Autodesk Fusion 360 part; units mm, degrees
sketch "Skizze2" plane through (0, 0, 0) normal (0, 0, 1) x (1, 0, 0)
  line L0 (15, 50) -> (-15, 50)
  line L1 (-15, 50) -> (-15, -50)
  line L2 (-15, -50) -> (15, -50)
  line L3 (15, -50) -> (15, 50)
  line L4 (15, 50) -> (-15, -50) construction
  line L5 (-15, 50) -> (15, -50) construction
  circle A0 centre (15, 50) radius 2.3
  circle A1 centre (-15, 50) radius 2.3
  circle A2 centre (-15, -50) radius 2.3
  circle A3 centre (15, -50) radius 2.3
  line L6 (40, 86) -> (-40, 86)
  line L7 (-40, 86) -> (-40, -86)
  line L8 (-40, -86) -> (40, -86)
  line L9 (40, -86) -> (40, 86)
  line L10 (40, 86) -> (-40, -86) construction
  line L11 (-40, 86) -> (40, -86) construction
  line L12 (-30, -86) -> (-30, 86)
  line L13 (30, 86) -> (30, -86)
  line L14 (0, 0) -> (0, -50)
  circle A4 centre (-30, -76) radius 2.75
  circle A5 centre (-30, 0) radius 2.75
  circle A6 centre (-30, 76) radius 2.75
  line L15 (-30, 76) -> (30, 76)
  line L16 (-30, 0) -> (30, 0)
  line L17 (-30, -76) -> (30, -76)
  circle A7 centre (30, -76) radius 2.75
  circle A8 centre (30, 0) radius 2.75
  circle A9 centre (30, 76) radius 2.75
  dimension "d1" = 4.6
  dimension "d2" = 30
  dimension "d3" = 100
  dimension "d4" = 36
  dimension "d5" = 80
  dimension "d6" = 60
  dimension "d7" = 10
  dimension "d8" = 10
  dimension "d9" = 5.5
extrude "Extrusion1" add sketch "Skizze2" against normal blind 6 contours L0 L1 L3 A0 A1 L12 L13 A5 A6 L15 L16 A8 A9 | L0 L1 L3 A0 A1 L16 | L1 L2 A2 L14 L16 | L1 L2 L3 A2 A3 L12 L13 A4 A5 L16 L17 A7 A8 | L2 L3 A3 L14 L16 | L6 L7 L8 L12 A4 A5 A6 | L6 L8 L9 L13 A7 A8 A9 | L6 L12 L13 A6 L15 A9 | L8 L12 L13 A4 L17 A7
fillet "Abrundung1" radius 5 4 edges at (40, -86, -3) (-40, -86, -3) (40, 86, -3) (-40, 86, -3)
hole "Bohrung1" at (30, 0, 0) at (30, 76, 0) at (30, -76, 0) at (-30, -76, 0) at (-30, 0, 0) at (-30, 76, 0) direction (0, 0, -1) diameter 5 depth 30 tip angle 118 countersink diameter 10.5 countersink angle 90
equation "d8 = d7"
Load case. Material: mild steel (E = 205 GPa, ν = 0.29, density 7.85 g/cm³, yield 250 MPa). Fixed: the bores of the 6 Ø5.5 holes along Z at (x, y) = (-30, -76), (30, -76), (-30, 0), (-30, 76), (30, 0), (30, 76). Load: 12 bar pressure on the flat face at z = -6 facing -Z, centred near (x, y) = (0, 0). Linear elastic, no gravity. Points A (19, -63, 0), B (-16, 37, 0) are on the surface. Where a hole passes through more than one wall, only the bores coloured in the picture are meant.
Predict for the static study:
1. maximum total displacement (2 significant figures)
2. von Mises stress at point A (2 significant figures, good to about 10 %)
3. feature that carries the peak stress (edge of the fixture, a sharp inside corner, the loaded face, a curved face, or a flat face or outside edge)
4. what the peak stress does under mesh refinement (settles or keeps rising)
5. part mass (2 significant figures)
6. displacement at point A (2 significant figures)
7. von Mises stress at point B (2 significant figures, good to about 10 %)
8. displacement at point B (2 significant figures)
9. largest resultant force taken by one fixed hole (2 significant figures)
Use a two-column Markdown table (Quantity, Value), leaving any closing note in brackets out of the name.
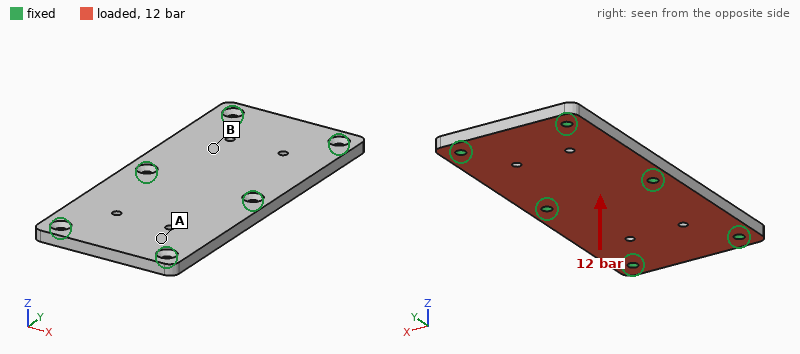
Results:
| Quantity | Value |
|---|---|
| maximum total displacement | 56 µm |
| von Mises stress at point A | 25 MPa |
| feature that carries the peak stress | edge of the fixture |
| what the peak stress does under mesh refinement | keeps rising |
| part mass | 630 g |
| displacement at point A | 28 µm |
| von Mises stress at point B | 50 MPa |
| displacement at point B | 50 µm |
| largest resultant force taken by one fixed hole | 4.0 kN |
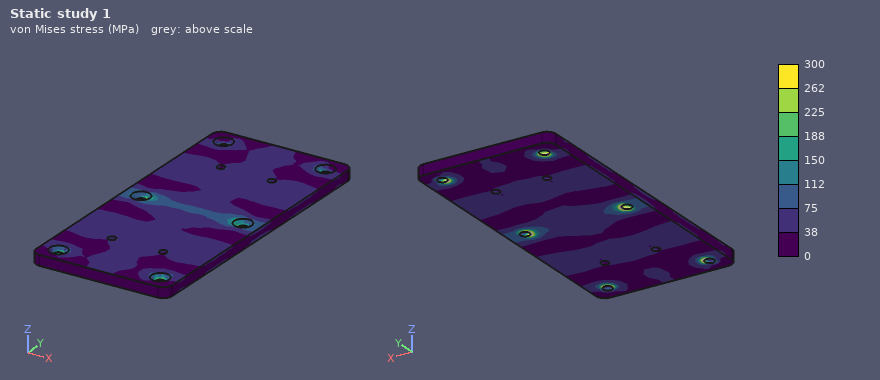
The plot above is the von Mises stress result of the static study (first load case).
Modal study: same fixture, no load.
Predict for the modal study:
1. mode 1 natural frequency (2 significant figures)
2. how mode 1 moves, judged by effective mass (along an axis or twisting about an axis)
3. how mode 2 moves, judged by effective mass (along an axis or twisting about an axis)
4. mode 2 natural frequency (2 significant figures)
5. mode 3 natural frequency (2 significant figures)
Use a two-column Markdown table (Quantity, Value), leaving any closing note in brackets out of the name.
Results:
| Quantity | Value |
|---|---|
| mode 1 natural frequency | 3800 Hz |
| how mode 1 moves, judged by effective mass | twisting about X |
| how mode 2 moves, judged by effective mass | along Z |
| mode 2 natural frequency | 4000 Hz |
| mode 3 natural frequency | 5400 Hz |
